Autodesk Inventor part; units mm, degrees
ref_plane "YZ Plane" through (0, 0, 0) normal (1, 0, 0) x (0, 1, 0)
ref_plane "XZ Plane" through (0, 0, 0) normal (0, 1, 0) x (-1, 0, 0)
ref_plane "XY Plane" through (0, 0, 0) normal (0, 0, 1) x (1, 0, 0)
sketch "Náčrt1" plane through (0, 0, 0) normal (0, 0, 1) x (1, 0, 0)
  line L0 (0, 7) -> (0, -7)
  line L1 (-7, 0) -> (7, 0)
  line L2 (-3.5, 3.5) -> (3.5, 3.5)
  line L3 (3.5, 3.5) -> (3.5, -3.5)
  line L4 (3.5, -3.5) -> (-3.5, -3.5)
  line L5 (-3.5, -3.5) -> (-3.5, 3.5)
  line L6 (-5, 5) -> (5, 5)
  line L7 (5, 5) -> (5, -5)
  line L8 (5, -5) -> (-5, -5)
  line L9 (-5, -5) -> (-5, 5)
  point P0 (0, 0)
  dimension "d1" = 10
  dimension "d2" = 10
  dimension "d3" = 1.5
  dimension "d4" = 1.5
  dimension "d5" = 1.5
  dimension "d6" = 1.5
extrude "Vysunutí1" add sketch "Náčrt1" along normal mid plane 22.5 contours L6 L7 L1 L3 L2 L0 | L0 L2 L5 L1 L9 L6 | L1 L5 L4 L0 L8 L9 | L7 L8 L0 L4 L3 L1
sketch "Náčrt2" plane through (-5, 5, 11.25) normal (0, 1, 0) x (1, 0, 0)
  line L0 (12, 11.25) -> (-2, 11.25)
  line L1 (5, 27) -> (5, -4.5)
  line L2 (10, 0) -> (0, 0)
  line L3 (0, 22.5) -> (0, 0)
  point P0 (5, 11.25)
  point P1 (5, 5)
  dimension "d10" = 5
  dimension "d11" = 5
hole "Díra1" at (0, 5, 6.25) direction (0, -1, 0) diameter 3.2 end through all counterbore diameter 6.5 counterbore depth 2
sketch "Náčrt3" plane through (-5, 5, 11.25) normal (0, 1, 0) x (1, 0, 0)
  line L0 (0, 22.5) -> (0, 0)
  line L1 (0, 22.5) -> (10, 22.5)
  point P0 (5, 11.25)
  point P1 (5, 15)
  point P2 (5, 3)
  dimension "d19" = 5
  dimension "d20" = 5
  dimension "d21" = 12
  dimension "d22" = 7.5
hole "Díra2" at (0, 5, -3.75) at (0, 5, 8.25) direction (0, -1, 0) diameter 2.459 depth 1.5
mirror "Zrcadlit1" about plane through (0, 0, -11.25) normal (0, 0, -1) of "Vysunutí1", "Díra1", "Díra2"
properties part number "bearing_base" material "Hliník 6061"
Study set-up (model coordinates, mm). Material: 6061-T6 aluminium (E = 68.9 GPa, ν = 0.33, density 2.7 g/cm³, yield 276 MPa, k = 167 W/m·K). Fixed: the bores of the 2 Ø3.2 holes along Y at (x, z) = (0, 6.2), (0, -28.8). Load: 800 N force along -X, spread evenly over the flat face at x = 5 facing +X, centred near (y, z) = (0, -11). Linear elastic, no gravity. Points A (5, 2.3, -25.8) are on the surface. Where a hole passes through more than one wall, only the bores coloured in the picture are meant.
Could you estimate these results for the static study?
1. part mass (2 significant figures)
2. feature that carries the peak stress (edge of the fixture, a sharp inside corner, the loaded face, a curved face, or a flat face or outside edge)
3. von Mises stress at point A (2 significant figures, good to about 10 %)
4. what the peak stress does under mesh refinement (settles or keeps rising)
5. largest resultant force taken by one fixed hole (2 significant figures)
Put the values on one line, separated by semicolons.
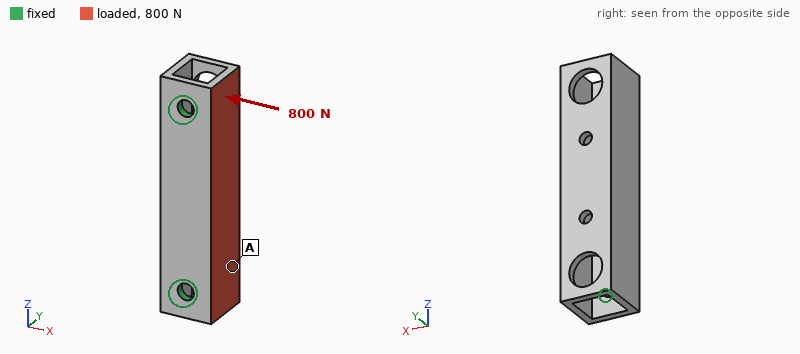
5.8 g; edge of the fixture; 35 MPa; keeps rising; 400 N
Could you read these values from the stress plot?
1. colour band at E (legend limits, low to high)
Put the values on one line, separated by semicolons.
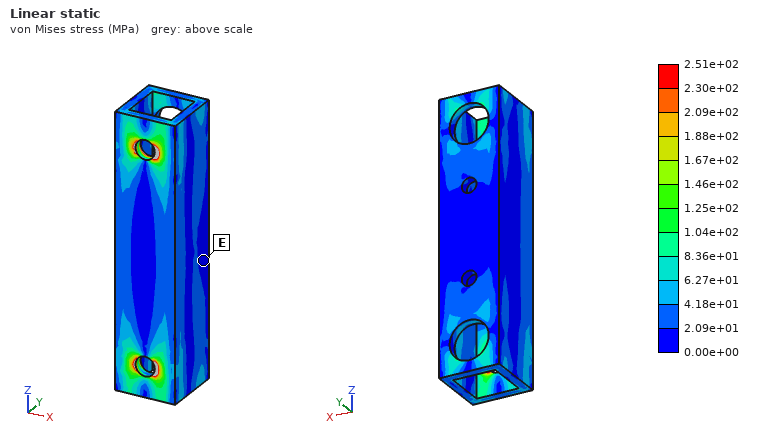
0.00e+00 to 2.09e+01 MPa
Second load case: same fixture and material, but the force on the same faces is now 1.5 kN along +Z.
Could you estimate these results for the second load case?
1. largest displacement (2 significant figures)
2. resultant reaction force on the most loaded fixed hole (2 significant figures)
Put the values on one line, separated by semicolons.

21 µm; 790 N
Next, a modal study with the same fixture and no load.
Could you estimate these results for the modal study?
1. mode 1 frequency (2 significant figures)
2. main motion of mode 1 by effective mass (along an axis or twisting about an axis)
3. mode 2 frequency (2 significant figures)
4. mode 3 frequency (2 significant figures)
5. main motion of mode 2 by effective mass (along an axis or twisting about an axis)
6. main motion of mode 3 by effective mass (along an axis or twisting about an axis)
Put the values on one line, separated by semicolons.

6900 Hz; along X; 16 kHz; 20 kHz; along Y; twisting about Y
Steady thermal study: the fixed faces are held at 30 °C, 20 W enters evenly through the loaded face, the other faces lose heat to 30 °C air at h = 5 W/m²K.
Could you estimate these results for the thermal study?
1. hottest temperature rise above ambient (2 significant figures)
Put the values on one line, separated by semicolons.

20 K
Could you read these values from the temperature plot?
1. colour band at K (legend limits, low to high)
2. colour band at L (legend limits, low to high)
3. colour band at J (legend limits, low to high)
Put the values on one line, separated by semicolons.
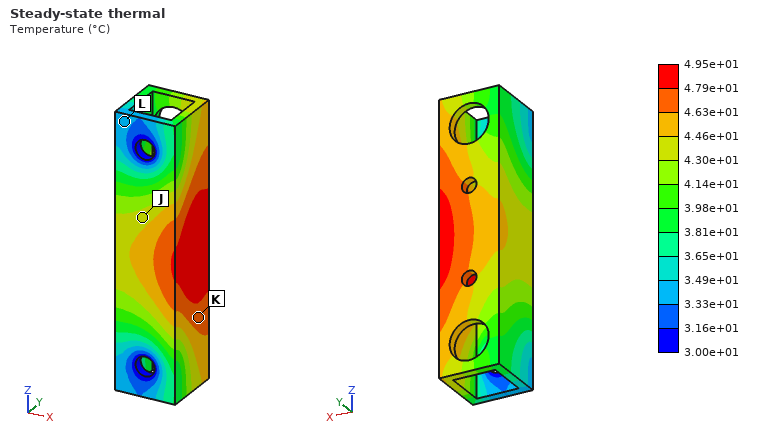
4.63e+01 to 4.79e+01 °C; 3.33e+01 to 3.49e+01 °C; 4.30e+01 to 4.46e+01 °C
